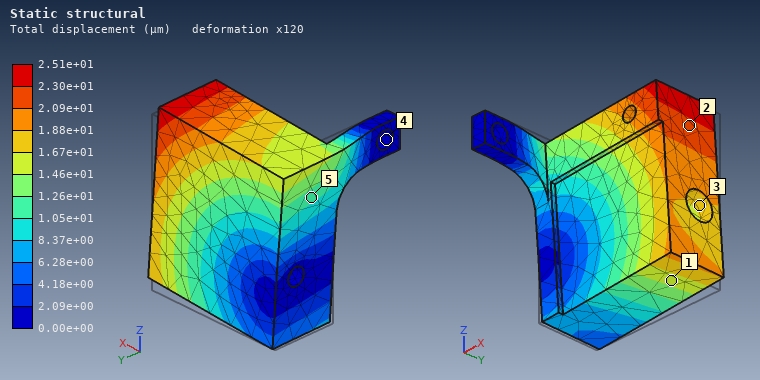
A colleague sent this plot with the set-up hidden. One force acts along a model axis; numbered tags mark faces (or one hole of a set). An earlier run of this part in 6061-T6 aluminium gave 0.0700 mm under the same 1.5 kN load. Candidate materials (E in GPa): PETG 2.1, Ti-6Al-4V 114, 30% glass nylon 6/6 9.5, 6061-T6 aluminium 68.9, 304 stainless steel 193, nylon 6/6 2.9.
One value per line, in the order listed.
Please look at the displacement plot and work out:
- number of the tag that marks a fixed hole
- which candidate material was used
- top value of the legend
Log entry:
4
304 stainless steel
2.51e+01 µm
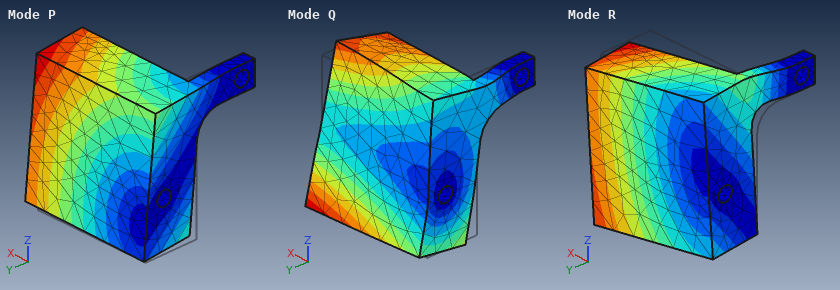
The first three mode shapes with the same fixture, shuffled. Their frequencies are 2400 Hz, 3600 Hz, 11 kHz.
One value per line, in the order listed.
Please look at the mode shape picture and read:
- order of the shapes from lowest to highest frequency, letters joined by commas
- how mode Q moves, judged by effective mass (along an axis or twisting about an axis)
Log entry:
P, R, Q
twisting about X
